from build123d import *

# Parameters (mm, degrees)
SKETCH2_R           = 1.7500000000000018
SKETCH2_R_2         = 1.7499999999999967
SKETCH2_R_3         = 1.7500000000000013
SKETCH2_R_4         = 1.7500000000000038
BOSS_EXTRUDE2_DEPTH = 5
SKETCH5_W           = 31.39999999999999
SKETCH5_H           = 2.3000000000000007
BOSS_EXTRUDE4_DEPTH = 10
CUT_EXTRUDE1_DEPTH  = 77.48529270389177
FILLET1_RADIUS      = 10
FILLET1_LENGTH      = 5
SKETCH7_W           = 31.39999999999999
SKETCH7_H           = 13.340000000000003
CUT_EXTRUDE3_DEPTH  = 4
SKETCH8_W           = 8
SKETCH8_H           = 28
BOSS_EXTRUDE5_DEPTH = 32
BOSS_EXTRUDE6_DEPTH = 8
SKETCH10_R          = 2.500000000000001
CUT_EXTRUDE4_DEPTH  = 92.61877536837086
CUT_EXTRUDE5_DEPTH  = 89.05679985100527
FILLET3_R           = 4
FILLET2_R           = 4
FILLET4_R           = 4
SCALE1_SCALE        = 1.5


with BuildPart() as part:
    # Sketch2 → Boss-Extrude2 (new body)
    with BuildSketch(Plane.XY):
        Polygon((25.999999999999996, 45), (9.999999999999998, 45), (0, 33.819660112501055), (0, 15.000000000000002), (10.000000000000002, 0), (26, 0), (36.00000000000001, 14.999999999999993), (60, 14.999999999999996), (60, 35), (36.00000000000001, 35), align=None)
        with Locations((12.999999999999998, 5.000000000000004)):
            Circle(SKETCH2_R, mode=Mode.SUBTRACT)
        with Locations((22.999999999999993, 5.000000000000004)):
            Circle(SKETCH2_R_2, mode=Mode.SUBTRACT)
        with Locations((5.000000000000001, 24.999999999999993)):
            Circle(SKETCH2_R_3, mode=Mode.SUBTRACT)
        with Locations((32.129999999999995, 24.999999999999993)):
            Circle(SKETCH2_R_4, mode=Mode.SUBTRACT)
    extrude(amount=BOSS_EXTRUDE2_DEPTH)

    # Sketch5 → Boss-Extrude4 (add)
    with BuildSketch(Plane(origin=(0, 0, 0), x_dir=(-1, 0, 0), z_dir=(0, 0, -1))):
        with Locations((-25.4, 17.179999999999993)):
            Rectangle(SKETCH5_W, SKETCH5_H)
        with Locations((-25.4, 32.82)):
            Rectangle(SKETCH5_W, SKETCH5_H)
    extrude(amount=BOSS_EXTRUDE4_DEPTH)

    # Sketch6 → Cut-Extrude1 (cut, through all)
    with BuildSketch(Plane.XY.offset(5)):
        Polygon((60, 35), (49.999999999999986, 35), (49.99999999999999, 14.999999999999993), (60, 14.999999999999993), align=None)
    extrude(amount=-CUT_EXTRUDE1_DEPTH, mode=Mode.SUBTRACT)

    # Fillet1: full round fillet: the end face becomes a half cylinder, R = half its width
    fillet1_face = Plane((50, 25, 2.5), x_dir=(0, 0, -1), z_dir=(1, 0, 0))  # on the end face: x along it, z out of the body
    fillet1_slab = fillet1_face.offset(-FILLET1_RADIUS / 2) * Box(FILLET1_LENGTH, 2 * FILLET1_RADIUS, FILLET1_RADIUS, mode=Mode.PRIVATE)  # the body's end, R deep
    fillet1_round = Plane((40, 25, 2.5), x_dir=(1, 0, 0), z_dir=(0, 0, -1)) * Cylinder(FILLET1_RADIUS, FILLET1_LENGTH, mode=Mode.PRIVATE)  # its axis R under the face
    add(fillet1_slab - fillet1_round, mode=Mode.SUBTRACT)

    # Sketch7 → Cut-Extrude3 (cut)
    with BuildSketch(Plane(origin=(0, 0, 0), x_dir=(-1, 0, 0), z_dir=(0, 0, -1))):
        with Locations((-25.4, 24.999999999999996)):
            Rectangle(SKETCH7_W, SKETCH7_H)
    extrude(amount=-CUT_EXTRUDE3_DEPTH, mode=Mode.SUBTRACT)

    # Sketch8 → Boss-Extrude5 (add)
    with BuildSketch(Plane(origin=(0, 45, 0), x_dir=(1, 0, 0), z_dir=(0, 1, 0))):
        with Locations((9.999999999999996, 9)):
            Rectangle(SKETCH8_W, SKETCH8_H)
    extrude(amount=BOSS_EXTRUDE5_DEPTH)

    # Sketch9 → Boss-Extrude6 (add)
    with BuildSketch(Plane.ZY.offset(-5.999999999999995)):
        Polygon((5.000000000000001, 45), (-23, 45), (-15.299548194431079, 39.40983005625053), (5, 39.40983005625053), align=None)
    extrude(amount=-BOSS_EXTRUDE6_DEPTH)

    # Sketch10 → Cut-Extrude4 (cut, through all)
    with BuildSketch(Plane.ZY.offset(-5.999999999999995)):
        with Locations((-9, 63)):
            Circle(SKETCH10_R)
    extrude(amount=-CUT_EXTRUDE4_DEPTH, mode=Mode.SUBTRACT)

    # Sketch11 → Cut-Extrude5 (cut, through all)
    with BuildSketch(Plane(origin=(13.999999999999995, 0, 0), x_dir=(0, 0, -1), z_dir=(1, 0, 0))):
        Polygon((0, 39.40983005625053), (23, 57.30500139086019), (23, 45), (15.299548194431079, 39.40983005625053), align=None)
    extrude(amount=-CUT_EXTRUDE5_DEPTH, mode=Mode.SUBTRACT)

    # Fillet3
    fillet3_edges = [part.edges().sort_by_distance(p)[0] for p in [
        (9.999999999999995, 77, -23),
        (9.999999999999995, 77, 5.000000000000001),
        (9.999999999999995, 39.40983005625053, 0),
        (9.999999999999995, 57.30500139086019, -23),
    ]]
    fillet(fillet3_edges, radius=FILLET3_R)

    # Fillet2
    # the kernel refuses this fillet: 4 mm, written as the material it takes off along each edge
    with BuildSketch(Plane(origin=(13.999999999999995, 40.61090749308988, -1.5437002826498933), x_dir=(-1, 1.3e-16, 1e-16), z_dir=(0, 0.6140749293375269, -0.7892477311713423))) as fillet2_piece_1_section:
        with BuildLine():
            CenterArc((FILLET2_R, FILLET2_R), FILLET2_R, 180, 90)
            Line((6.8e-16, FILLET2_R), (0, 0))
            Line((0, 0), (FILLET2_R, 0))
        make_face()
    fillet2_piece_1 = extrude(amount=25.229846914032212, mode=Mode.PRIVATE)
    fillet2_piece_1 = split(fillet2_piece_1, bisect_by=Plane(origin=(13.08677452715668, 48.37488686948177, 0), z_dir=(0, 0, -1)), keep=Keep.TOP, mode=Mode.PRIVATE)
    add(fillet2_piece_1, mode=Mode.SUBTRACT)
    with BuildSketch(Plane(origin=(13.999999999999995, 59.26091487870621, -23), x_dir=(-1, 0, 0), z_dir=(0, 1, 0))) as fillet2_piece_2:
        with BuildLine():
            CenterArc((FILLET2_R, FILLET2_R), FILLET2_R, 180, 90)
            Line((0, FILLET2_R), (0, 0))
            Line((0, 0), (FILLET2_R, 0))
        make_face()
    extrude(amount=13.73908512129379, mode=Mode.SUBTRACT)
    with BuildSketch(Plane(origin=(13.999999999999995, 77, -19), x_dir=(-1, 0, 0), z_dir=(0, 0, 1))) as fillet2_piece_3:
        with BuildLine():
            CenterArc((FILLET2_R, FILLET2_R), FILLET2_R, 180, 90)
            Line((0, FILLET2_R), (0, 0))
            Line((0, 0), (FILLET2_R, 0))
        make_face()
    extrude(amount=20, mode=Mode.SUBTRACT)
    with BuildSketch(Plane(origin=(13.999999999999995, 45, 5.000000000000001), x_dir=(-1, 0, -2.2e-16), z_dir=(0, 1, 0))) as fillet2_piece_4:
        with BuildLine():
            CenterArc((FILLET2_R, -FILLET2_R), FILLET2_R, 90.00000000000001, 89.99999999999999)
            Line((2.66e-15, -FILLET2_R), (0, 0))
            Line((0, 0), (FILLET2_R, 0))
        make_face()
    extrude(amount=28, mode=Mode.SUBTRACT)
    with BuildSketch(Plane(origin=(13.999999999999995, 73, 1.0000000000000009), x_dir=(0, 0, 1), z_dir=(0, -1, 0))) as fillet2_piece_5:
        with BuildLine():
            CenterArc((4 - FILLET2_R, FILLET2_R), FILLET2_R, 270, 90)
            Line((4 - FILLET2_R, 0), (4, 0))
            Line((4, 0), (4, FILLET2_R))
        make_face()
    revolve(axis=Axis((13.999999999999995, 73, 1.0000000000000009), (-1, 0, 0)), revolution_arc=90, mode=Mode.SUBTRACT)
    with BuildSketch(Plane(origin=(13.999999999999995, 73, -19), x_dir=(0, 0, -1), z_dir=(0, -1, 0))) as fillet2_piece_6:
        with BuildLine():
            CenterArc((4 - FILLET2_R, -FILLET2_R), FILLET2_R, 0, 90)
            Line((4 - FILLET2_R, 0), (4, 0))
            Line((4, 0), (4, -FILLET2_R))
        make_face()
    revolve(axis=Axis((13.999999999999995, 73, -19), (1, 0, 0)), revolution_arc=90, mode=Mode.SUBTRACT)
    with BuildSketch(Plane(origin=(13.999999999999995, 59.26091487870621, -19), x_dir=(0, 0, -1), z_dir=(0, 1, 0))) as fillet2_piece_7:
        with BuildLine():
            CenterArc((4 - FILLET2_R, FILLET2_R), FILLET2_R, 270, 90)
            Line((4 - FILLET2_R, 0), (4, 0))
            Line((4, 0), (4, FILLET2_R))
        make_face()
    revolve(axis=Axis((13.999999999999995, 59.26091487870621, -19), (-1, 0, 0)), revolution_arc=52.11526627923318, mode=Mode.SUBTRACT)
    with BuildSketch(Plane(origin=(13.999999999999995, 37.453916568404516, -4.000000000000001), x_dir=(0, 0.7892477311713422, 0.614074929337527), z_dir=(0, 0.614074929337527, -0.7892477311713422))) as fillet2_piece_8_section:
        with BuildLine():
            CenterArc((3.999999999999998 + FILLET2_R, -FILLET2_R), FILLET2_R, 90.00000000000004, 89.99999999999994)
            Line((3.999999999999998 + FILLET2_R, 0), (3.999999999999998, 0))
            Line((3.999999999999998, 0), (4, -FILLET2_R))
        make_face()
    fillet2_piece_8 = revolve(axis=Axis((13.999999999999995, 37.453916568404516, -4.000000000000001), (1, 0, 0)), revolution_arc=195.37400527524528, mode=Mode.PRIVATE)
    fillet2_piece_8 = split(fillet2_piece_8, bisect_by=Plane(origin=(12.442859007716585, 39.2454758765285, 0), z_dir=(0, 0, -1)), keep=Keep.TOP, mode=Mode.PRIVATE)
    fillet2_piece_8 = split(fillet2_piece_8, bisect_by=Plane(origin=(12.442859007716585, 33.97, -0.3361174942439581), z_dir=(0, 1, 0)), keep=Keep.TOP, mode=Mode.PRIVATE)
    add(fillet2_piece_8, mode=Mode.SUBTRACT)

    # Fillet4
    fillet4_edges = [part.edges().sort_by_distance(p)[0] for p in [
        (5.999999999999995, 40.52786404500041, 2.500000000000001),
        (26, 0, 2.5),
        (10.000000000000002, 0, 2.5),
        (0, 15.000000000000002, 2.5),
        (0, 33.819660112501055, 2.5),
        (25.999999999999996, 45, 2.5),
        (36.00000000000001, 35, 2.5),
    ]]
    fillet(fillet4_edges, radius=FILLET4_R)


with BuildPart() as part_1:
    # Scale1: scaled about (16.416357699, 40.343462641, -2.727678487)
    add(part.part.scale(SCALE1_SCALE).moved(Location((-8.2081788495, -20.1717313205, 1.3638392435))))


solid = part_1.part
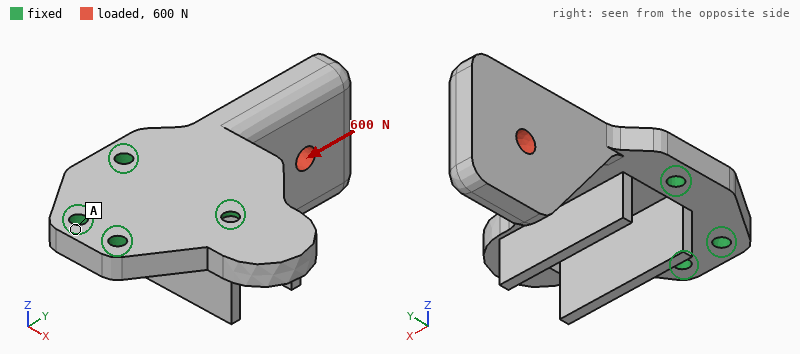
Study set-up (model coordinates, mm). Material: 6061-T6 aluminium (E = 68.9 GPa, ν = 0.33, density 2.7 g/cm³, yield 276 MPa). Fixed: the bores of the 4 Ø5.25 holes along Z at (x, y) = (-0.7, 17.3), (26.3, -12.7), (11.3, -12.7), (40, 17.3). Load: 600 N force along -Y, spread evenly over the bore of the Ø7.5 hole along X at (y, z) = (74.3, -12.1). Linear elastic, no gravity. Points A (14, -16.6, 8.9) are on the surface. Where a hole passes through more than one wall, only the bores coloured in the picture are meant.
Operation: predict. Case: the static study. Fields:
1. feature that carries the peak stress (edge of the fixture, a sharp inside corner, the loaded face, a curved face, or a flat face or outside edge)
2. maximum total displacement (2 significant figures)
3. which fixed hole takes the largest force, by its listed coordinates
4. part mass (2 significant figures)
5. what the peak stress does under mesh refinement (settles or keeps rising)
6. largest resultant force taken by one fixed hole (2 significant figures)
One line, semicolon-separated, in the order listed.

edge of the fixture; 0.45 mm; (-0.7, 17.3); 120 g; keeps rising; 670 N
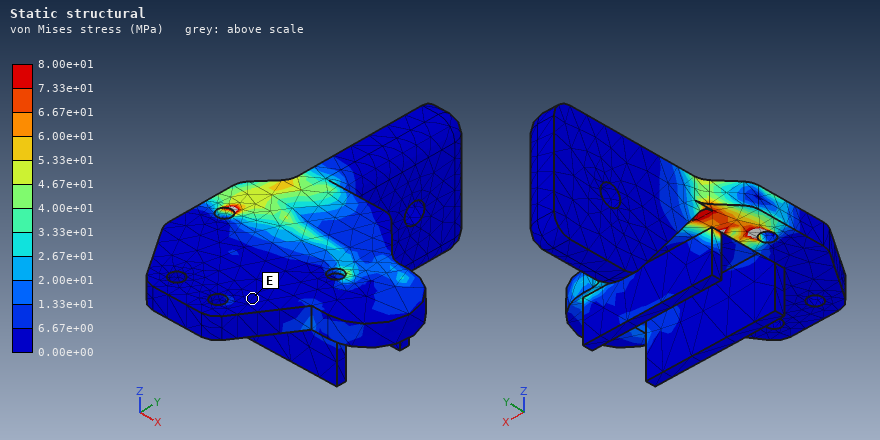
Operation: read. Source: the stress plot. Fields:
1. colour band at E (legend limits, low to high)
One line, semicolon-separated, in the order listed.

0.00e+00 to 6.67e+00 MPa
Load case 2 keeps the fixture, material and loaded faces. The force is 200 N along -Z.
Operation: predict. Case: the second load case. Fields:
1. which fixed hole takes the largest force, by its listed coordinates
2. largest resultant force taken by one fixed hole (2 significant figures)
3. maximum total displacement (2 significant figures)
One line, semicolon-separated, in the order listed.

(-0.7, 17.3); 320 N; 0.37 mm
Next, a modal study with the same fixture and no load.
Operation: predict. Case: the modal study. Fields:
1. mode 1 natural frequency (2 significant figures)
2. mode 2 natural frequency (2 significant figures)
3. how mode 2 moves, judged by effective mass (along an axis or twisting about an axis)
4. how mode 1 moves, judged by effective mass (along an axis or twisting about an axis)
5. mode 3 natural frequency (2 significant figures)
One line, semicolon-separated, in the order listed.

580 Hz; 1400 Hz; along X; along Z; 2900 Hz
